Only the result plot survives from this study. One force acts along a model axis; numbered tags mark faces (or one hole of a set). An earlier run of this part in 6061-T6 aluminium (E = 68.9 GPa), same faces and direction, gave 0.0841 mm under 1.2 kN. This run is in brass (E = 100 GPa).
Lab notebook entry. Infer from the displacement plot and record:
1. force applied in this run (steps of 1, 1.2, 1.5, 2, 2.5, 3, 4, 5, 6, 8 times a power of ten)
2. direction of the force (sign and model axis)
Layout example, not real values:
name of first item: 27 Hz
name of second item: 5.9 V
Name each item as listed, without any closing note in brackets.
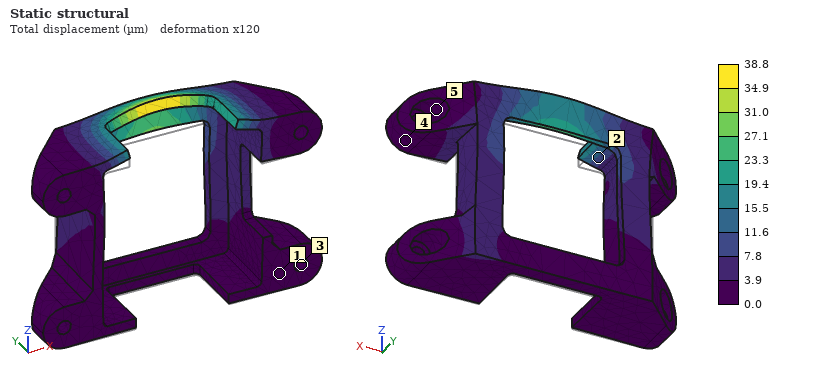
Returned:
force applied in this run: 800 N
direction of the force: +Z
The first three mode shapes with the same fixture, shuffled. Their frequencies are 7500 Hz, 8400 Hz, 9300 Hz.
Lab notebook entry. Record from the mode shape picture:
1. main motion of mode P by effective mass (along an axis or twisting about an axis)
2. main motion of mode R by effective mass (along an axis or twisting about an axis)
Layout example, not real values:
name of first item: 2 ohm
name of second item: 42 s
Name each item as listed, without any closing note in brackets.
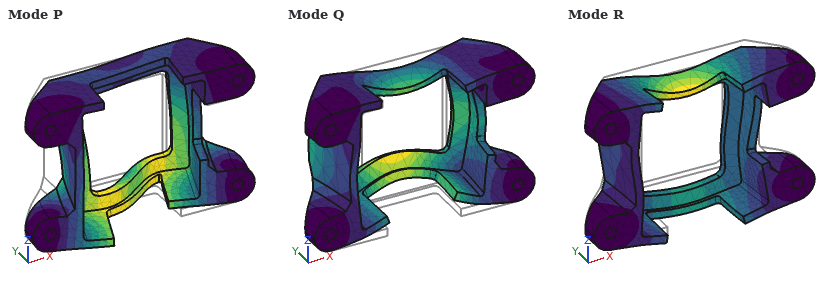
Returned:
main motion of mode P by effective mass: along X
main motion of mode R by effective mass: along Z
